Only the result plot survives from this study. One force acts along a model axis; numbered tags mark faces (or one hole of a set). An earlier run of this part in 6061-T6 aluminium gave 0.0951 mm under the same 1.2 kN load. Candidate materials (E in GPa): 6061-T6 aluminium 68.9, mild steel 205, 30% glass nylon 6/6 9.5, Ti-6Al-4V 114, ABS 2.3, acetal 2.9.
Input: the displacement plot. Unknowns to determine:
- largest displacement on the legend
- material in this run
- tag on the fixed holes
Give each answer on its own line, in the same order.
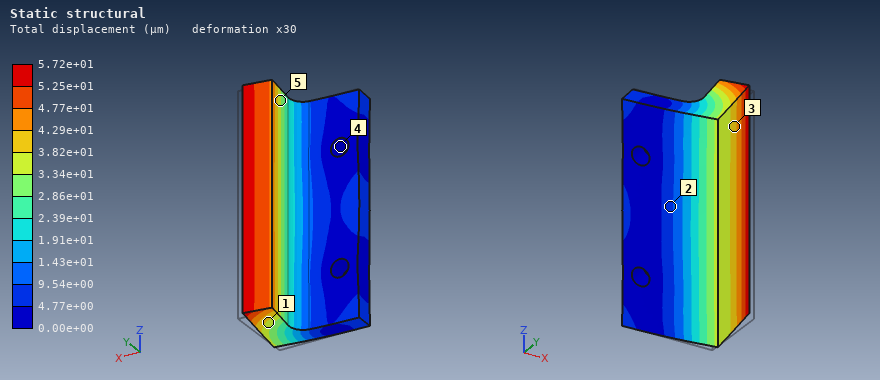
5.72e+01 µm
Ti-6Al-4V
4
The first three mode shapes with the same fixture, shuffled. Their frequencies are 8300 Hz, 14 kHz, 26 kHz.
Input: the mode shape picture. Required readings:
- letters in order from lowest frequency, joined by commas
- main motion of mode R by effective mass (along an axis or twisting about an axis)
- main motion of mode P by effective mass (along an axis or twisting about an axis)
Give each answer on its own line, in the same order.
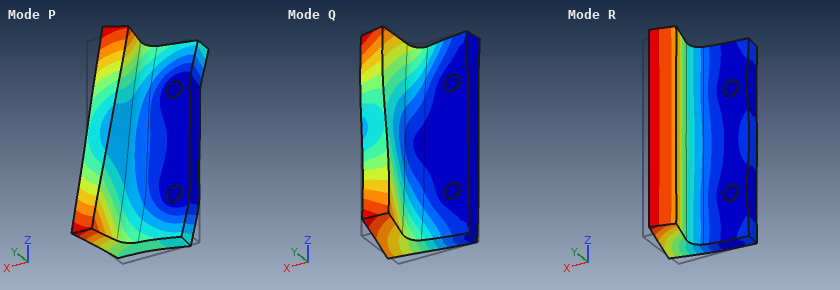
R, Q, P
along Y
along Z
